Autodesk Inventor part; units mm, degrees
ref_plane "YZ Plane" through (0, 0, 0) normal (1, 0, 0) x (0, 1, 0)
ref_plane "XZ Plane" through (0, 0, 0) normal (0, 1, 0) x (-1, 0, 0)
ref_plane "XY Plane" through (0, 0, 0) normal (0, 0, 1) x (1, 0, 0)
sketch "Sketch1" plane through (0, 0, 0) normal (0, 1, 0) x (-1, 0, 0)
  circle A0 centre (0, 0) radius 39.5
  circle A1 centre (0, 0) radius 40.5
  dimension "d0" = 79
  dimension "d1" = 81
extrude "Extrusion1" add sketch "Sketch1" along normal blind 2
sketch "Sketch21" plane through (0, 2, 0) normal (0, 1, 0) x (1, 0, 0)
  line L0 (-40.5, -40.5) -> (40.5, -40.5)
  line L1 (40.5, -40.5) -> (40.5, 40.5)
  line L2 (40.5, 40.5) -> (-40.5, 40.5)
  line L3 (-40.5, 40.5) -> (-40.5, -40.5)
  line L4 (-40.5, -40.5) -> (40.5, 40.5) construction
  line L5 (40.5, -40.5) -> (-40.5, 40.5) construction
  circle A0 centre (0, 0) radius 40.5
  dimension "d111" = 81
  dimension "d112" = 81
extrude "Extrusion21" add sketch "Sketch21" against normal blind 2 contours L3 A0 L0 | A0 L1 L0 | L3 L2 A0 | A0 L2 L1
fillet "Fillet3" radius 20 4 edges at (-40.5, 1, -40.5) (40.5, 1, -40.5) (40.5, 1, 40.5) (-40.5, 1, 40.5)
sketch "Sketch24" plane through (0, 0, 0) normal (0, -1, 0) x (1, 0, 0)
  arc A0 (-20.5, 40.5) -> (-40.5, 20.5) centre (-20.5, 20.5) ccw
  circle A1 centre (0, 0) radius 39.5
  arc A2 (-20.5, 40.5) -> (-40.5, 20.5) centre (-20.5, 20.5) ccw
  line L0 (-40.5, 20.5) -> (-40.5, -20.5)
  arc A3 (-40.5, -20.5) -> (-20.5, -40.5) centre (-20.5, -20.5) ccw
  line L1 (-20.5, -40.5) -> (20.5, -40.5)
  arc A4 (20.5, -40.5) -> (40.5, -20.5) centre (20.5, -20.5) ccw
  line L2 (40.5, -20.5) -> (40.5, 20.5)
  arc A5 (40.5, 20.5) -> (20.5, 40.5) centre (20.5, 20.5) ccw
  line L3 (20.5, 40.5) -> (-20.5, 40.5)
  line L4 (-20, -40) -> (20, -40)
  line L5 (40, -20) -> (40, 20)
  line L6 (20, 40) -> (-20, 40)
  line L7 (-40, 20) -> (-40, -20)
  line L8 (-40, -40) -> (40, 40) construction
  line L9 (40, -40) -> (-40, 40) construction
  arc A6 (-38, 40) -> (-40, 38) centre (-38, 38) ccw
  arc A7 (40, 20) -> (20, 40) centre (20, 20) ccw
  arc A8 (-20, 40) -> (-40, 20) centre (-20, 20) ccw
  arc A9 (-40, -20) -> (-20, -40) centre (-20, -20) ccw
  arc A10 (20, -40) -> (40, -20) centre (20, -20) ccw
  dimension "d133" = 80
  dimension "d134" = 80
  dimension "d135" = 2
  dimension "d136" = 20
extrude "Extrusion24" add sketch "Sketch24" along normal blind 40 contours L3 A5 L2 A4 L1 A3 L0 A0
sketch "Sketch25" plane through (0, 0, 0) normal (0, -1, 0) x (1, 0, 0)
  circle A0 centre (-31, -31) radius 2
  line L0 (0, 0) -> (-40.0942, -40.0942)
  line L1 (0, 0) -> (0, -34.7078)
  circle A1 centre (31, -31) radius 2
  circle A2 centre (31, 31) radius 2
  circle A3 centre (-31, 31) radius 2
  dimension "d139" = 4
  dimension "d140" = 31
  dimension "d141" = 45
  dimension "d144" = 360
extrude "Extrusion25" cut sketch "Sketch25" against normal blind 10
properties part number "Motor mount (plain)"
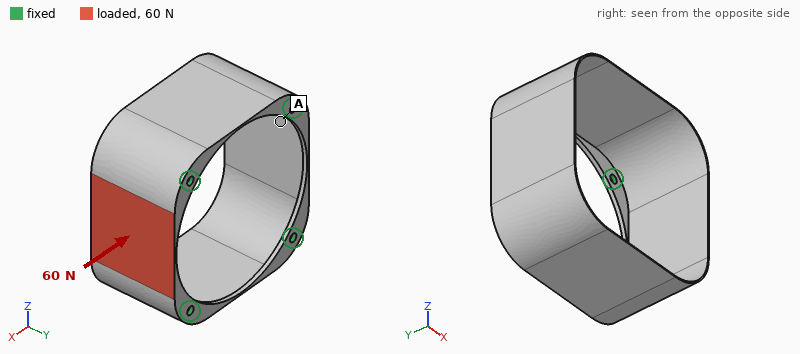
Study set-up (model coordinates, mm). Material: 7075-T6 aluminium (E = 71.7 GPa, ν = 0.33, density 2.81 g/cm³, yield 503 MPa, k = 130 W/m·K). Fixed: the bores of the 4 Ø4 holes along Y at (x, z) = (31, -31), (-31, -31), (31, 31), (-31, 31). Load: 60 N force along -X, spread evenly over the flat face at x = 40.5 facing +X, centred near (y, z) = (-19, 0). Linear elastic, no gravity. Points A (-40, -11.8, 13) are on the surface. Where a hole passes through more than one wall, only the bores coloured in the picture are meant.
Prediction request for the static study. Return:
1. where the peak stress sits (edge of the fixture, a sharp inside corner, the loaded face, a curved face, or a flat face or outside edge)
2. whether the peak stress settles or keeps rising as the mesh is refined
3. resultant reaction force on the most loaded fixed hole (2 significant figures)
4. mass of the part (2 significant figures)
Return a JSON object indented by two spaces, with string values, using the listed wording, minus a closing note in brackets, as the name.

{
  "where the peak stress sits": "edge of the fixture",
  "whether the peak stress settles or keeps rising as the mesh is refined": "keeps rising",
  "resultant reaction force on the most loaded fixed hole": "58 N",
  "mass of the part": "25 g"
}
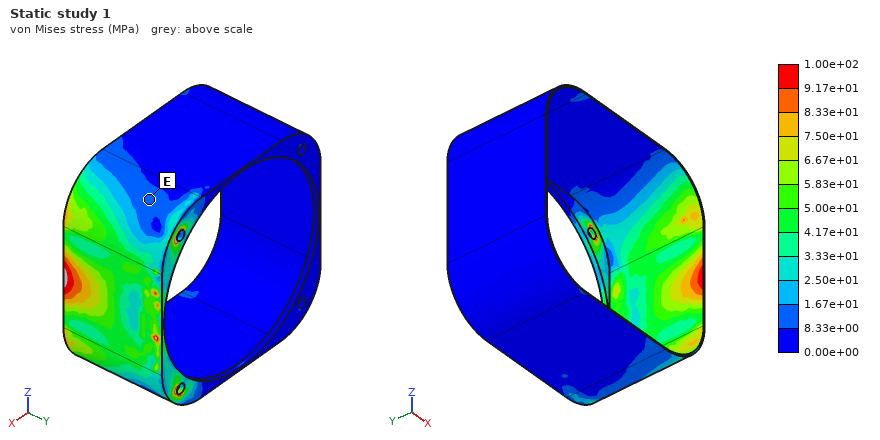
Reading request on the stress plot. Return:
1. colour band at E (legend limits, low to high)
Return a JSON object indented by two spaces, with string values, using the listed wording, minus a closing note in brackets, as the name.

{
  "colour band at E": "8.33e+00 to 1.67e+01 MPa"
}
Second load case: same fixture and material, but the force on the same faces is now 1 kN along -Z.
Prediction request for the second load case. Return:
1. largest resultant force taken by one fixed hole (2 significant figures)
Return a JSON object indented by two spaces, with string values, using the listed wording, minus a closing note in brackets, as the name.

{
  "largest resultant force taken by one fixed hole": "600 N"
}
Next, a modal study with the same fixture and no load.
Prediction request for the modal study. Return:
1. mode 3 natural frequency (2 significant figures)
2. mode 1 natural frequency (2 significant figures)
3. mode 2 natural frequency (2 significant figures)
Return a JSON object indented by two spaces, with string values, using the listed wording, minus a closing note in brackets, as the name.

{
  "mode 3 natural frequency": "830 Hz",
  "mode 1 natural frequency": "770 Hz",
  "mode 2 natural frequency": "830 Hz"
}
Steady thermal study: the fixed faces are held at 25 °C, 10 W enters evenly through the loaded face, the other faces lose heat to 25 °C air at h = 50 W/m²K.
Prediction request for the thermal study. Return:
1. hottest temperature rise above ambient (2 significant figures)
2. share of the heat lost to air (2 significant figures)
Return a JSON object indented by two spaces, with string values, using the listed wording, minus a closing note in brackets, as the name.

{
  "hottest temperature rise above ambient": "32 K",
  "share of the heat lost to air": "52 %"
}
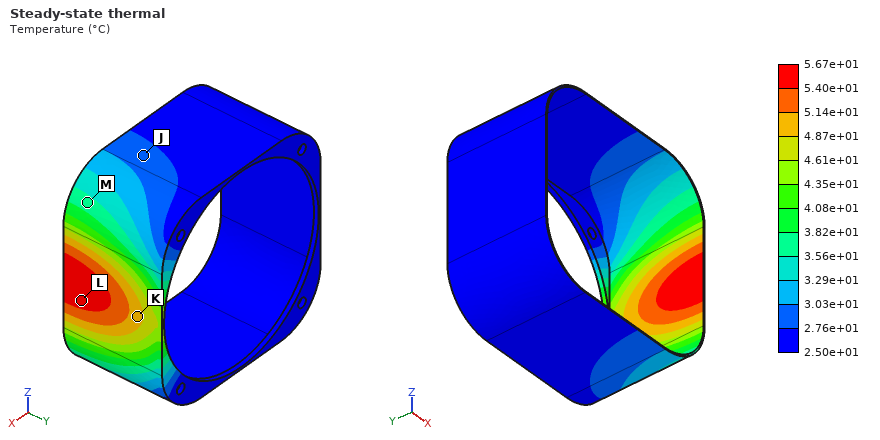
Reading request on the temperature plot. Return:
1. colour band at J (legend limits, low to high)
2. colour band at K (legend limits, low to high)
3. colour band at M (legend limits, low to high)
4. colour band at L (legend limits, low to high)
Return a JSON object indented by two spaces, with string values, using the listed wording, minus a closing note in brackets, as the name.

{
  "colour band at J": "2.76e+01 to 3.03e+01 °C",
  "colour band at K": "4.87e+01 to 5.14e+01 °C",
  "colour band at M": "3.56e+01 to 3.82e+01 °C",
  "colour band at L": "5.40e+01 to 5.67e+01 °C"
}
